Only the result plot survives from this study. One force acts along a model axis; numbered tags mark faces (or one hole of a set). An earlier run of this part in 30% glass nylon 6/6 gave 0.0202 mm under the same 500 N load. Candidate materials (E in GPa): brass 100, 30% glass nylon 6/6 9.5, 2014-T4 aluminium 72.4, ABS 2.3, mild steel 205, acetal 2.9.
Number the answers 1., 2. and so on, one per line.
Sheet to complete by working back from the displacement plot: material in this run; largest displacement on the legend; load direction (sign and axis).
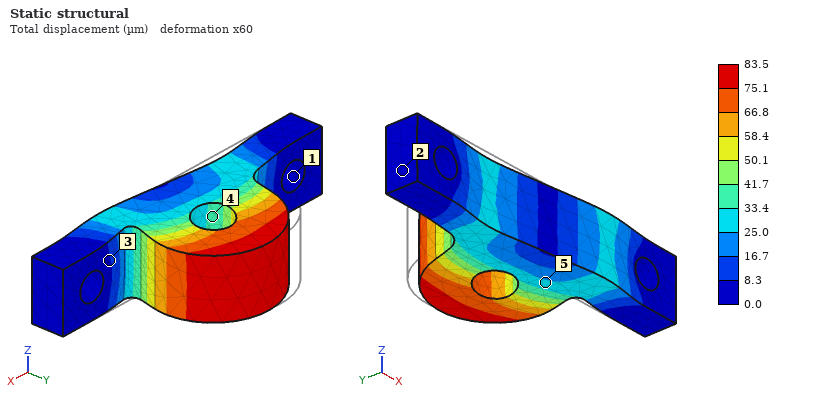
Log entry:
1. ABS
2. 83.5 µm
3. +X
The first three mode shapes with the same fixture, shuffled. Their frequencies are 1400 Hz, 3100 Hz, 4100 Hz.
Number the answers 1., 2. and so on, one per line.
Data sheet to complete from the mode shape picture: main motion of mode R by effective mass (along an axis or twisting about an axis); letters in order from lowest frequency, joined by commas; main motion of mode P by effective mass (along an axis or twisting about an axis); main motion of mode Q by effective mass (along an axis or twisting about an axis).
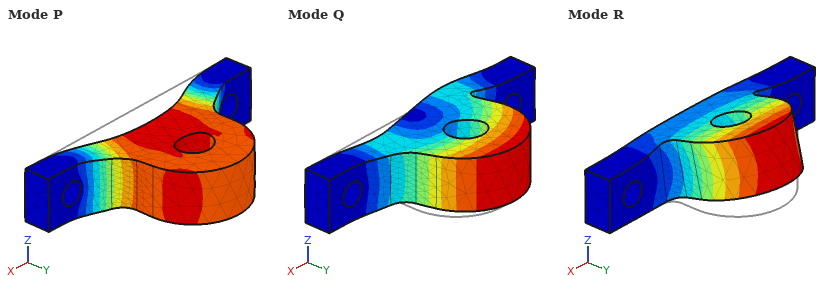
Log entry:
1. along Z
2. R, P, Q
3. along Y
4. along X
